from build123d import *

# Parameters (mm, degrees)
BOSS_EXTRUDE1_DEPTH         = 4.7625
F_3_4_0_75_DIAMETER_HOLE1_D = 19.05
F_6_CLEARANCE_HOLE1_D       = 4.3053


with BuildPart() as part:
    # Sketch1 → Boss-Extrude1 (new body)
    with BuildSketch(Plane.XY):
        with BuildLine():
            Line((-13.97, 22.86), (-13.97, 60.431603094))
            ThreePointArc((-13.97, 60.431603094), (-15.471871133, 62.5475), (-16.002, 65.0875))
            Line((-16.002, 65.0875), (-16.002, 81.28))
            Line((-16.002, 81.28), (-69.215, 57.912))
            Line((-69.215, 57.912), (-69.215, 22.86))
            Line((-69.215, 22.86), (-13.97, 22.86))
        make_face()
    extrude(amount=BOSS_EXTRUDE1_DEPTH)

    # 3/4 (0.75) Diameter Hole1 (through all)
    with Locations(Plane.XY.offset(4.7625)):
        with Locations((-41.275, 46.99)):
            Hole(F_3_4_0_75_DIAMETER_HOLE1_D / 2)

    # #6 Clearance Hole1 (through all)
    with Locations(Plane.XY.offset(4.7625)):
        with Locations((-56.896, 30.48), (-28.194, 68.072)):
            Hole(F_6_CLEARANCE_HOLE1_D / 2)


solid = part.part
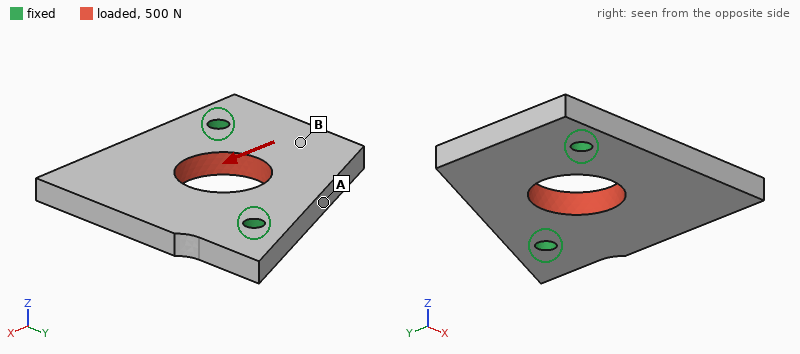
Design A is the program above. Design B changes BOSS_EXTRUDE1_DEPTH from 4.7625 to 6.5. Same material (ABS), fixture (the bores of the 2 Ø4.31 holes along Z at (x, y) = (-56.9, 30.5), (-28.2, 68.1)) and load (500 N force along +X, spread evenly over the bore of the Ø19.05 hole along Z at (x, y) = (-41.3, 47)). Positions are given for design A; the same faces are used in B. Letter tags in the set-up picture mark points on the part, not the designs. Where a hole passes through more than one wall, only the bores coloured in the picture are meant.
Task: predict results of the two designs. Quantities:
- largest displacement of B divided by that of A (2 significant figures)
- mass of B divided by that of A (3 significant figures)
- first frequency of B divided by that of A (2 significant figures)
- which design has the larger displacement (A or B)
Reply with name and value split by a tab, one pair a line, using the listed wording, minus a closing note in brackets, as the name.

largest displacement of B divided by that of A	0.73
mass of B divided by that of A	1.36
first frequency of B divided by that of A	1.3
which design has the larger displacement	A
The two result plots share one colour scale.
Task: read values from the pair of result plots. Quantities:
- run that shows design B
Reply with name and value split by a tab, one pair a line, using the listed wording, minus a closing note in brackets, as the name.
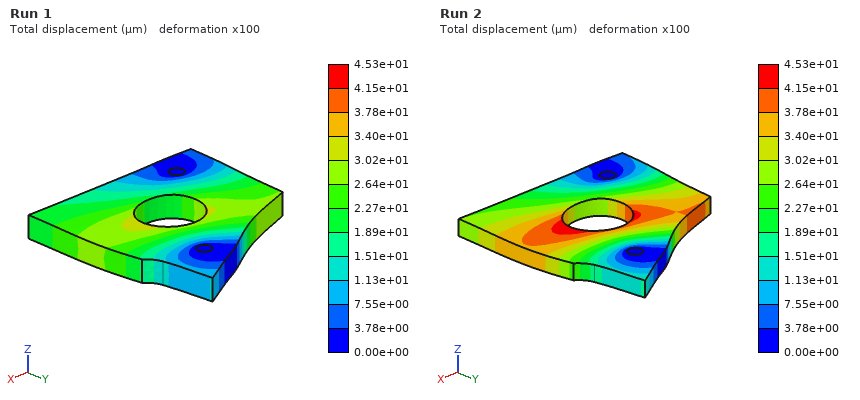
run that shows design B	Run 1
